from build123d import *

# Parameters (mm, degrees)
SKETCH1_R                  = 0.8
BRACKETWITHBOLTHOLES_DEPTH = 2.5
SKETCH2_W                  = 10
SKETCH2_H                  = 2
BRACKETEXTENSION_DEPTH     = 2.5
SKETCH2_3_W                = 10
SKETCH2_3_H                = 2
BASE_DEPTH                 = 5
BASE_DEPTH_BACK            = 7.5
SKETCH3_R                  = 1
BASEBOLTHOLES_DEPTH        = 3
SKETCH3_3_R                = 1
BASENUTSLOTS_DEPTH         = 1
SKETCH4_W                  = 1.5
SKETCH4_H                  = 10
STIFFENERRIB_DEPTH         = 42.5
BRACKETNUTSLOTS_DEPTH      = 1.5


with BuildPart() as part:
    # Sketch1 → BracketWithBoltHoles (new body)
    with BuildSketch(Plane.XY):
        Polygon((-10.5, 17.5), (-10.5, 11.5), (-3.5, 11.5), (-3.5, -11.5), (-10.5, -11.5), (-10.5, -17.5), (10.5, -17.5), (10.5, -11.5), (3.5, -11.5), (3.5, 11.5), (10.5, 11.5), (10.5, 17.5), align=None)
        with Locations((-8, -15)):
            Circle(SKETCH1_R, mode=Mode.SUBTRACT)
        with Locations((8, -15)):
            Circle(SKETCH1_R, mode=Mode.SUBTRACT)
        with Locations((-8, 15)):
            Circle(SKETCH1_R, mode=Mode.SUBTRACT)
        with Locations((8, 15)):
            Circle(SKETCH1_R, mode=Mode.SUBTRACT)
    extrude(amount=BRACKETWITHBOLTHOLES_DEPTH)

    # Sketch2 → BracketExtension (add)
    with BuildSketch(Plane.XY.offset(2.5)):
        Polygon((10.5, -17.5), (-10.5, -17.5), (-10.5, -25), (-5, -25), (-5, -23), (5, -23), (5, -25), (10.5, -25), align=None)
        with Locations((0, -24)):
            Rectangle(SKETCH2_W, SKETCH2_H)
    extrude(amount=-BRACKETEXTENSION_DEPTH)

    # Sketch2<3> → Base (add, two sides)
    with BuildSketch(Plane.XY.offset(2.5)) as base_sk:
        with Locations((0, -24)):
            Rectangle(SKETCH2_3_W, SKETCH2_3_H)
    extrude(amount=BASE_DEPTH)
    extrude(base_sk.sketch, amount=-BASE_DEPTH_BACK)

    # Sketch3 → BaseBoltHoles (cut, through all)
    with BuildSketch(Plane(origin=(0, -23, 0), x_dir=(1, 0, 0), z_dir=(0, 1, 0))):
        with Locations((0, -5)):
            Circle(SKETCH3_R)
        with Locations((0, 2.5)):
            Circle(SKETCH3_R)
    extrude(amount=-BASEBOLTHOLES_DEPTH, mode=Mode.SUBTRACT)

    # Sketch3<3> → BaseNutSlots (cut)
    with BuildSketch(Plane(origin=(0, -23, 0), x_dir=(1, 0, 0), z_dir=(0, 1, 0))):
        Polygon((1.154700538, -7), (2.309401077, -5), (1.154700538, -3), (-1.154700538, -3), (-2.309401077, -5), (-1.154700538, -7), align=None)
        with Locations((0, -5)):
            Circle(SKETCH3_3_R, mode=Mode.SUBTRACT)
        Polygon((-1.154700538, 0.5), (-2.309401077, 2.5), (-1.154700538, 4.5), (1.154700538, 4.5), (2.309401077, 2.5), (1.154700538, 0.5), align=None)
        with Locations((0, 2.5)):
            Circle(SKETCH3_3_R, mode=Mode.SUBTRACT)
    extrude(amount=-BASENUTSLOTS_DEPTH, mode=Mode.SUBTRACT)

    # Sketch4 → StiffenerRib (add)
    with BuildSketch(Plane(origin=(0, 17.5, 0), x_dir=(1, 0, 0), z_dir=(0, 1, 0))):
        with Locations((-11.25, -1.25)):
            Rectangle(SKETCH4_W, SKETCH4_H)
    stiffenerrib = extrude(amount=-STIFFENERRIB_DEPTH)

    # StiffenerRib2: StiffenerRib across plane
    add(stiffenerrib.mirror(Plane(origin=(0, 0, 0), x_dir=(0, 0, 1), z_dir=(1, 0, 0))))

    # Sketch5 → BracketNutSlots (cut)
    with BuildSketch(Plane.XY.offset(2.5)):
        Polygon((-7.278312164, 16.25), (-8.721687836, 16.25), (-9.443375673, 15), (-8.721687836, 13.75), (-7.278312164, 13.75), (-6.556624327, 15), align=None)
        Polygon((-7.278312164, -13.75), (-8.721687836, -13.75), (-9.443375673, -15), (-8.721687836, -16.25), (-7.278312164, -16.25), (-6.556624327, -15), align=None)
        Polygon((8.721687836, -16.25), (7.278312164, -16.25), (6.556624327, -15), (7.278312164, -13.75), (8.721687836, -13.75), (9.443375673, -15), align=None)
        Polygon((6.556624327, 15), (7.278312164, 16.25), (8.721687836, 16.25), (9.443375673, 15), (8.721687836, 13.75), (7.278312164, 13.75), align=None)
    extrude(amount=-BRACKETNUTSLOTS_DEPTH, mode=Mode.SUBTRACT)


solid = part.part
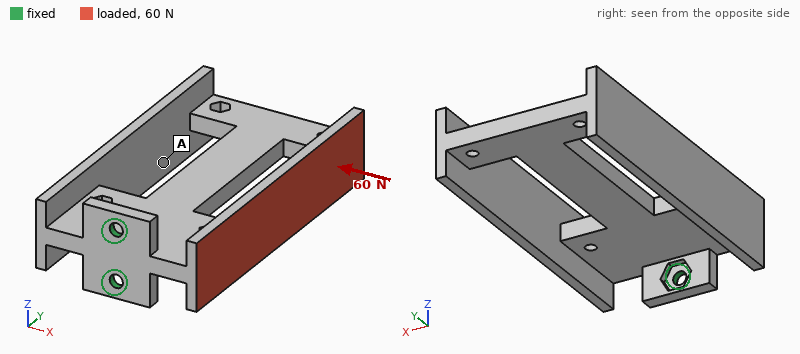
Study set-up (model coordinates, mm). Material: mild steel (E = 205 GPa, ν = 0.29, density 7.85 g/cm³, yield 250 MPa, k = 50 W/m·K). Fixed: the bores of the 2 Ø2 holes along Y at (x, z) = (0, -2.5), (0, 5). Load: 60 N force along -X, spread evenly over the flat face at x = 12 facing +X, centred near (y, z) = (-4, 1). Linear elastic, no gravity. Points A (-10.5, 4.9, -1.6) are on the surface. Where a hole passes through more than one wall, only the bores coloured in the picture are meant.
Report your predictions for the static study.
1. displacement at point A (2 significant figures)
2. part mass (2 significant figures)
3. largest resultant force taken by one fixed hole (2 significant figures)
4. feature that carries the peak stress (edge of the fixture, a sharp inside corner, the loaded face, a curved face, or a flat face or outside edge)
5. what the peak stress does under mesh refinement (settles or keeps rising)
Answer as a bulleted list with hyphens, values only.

- 69 µm
- 22 g
- 30 N
- edge of the fixture
- keeps rising
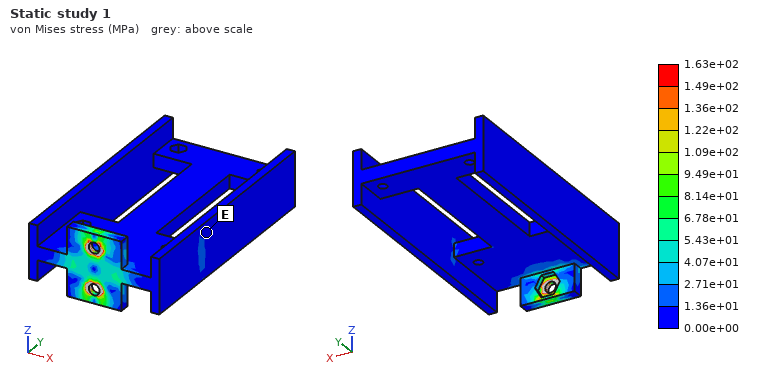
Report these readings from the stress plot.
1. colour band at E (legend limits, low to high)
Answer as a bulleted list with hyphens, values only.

- 0.00e+00 to 1.36e+01 MPa
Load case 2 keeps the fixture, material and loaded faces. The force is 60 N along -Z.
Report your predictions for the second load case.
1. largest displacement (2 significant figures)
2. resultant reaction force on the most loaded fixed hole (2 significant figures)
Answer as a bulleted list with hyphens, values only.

- 0.11 mm
- 210 N
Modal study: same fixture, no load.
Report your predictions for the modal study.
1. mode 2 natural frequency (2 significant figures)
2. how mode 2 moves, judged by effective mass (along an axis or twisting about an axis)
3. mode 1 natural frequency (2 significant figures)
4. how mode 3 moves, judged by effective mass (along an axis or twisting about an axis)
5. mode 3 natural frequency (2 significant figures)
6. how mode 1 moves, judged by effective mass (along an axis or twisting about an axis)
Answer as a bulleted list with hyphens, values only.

- 1200 Hz
- along Z
- 1000 Hz
- twisting about Y
- 2600 Hz
- along X
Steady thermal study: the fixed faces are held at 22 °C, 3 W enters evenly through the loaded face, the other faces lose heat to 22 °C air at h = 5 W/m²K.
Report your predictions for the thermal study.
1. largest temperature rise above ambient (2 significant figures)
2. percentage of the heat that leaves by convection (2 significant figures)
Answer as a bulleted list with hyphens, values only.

- 43 K
- 11 %
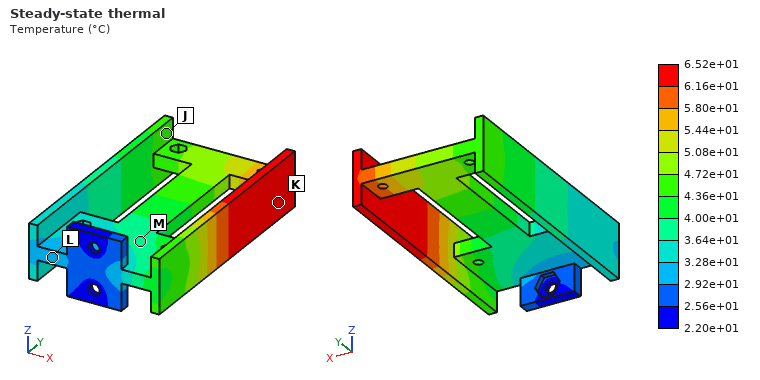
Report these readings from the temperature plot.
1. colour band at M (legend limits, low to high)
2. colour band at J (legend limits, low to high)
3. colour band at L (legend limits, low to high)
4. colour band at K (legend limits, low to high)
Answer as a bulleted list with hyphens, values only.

- 3.64e+01 to 4.00e+01 °C
- 4.36e+01 to 4.72e+01 °C
- 2.92e+01 to 3.28e+01 °C
- 6.16e+01 to 6.52e+01 °C
